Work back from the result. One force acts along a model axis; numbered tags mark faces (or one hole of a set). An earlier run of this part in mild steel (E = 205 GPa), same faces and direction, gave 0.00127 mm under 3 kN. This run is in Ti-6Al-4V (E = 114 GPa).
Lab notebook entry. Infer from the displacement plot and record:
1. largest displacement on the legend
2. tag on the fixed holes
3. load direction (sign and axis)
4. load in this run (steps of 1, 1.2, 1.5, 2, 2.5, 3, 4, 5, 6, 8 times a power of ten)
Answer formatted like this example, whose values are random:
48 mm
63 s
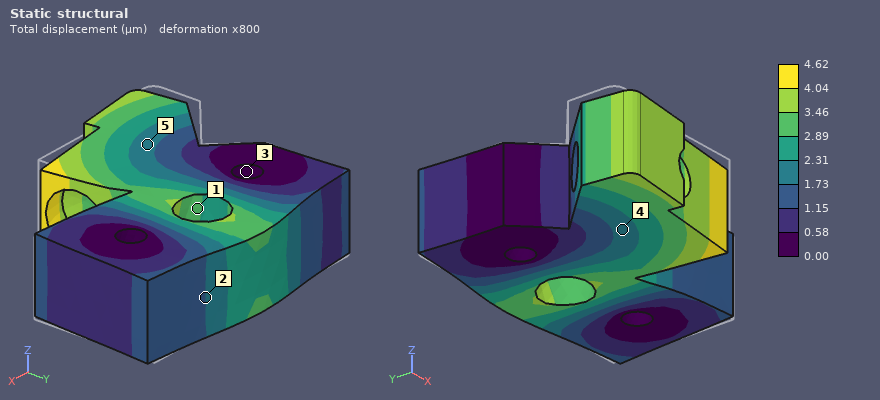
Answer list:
4.62 µm
3
+Y
6 kN
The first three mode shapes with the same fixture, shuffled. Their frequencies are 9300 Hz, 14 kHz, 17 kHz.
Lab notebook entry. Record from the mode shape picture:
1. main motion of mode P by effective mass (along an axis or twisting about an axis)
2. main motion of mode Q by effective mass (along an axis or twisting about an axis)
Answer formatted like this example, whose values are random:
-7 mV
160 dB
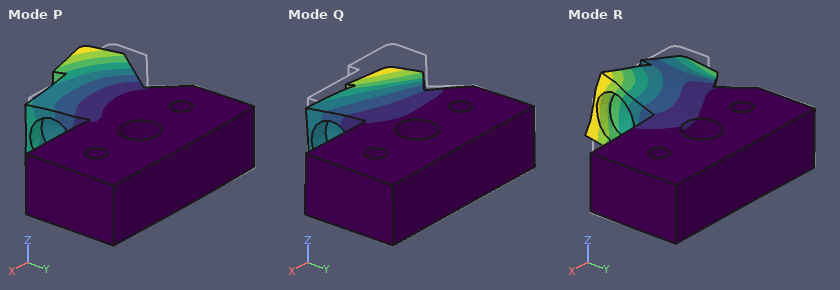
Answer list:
along X
along Z
